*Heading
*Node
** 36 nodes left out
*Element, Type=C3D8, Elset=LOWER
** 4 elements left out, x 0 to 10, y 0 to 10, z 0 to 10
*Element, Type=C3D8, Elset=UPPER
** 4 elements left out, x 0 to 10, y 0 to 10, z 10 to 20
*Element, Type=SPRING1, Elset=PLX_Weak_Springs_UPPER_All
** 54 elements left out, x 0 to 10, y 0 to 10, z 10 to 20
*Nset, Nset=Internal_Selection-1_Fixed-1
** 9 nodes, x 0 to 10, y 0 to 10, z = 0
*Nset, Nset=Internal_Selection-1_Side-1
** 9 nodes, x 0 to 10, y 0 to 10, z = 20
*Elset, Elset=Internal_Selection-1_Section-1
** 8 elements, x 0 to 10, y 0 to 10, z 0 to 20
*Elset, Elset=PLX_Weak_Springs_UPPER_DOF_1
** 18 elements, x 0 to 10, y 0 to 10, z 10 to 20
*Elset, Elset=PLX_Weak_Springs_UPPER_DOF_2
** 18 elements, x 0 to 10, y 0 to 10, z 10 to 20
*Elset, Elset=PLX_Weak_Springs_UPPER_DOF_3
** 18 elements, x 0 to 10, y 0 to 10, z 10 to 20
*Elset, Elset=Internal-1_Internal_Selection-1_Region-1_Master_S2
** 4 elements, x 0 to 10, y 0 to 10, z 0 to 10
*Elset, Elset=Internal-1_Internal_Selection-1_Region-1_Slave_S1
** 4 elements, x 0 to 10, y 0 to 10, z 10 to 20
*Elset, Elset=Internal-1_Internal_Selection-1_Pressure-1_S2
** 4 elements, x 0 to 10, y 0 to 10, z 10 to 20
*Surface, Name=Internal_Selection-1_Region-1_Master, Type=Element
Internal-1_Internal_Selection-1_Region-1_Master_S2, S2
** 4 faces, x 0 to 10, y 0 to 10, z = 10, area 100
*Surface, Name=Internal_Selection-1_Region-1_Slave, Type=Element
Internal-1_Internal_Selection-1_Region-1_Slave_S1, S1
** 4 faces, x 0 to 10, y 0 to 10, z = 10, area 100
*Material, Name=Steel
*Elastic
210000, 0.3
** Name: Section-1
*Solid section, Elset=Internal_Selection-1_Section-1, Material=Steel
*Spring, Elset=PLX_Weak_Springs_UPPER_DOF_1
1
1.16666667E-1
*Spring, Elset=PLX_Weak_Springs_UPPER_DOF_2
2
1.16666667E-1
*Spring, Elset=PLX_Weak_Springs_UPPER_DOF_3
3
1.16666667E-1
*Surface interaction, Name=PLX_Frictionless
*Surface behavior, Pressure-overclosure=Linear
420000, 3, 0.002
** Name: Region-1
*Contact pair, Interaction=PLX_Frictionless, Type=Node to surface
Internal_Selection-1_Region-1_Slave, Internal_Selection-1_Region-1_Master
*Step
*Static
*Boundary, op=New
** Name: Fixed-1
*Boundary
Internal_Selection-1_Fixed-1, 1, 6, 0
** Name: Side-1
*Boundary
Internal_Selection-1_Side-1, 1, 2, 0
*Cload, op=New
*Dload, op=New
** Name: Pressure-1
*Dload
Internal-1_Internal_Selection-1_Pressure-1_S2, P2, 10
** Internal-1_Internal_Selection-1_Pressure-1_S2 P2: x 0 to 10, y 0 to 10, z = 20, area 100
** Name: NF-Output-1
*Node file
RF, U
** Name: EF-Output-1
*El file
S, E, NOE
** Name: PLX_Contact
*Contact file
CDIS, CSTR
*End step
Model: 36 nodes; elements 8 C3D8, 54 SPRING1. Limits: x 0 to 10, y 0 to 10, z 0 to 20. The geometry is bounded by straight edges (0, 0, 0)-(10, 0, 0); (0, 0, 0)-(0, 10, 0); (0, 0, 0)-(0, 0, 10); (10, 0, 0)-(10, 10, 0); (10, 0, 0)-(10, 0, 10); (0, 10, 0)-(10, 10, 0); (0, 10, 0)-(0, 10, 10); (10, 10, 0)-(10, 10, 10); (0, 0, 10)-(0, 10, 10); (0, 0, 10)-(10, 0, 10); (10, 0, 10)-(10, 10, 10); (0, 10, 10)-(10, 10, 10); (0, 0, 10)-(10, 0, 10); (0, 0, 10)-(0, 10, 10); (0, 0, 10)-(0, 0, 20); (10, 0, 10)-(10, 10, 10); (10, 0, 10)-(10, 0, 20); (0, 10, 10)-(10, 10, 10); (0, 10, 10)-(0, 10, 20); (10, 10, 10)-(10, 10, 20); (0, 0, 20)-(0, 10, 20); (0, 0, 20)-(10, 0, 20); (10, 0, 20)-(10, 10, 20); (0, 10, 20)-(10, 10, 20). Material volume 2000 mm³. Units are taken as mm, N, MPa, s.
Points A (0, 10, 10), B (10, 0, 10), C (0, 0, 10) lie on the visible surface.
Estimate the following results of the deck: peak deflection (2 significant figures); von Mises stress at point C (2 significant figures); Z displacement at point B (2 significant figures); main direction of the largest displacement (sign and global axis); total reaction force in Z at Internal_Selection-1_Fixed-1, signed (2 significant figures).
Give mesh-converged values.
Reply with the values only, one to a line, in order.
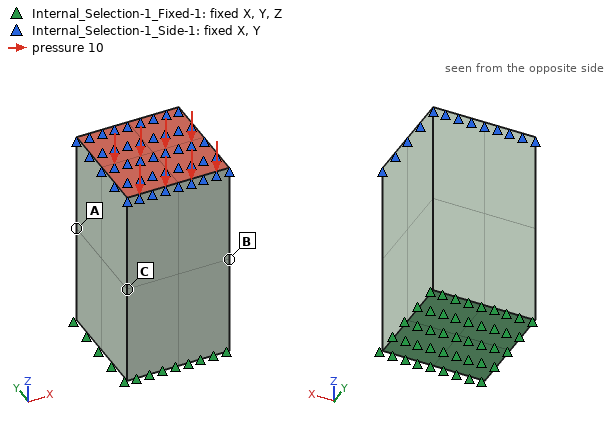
9.7e-04 mm
9.6 MPa
-4.8e-04 mm
-Z
1000 N
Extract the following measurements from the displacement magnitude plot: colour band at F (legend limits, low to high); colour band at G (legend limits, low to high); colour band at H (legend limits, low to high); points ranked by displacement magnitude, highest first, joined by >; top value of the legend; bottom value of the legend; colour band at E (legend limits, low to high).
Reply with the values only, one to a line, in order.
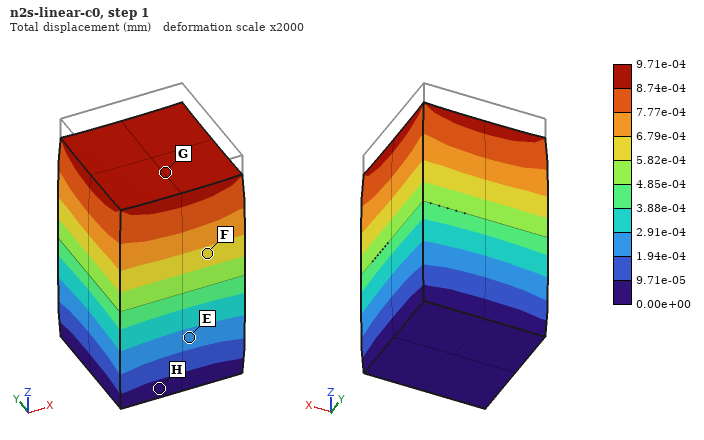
5.82e-04 to 6.79e-04 mm
8.74e-04 to 9.71e-04 mm
0.00e+00 to 9.71e-05 mm
G > F > E > H
9.71e-04 mm
0.00e+00 mm
1.94e-04 to 2.91e-04 mm
